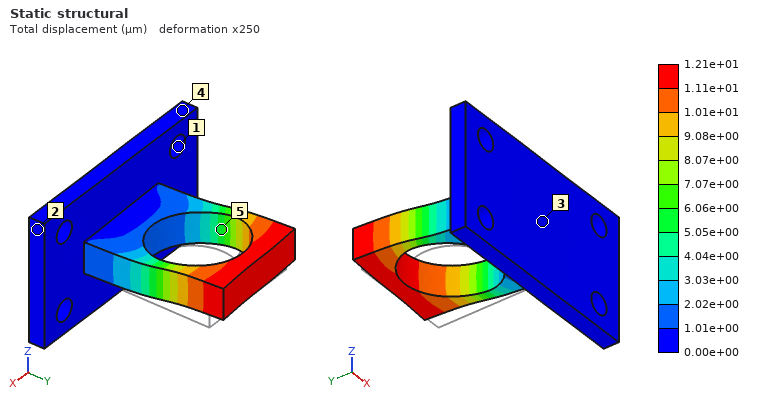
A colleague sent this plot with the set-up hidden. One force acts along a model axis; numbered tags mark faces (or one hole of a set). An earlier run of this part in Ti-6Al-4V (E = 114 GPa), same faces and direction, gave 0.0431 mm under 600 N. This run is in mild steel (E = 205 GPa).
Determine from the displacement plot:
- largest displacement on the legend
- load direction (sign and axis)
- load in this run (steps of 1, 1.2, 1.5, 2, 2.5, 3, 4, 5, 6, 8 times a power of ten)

1.21e+01 µm
-X
300 N
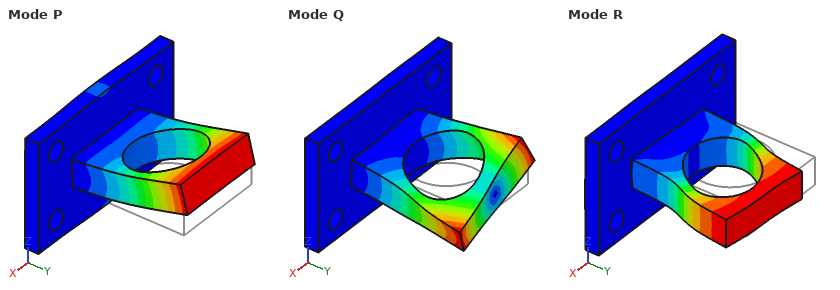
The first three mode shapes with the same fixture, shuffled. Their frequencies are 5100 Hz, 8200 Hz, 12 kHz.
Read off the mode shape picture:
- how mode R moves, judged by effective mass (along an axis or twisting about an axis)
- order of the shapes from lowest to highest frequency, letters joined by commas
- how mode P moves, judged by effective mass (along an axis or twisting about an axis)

along X
P, R, Q
along Z
